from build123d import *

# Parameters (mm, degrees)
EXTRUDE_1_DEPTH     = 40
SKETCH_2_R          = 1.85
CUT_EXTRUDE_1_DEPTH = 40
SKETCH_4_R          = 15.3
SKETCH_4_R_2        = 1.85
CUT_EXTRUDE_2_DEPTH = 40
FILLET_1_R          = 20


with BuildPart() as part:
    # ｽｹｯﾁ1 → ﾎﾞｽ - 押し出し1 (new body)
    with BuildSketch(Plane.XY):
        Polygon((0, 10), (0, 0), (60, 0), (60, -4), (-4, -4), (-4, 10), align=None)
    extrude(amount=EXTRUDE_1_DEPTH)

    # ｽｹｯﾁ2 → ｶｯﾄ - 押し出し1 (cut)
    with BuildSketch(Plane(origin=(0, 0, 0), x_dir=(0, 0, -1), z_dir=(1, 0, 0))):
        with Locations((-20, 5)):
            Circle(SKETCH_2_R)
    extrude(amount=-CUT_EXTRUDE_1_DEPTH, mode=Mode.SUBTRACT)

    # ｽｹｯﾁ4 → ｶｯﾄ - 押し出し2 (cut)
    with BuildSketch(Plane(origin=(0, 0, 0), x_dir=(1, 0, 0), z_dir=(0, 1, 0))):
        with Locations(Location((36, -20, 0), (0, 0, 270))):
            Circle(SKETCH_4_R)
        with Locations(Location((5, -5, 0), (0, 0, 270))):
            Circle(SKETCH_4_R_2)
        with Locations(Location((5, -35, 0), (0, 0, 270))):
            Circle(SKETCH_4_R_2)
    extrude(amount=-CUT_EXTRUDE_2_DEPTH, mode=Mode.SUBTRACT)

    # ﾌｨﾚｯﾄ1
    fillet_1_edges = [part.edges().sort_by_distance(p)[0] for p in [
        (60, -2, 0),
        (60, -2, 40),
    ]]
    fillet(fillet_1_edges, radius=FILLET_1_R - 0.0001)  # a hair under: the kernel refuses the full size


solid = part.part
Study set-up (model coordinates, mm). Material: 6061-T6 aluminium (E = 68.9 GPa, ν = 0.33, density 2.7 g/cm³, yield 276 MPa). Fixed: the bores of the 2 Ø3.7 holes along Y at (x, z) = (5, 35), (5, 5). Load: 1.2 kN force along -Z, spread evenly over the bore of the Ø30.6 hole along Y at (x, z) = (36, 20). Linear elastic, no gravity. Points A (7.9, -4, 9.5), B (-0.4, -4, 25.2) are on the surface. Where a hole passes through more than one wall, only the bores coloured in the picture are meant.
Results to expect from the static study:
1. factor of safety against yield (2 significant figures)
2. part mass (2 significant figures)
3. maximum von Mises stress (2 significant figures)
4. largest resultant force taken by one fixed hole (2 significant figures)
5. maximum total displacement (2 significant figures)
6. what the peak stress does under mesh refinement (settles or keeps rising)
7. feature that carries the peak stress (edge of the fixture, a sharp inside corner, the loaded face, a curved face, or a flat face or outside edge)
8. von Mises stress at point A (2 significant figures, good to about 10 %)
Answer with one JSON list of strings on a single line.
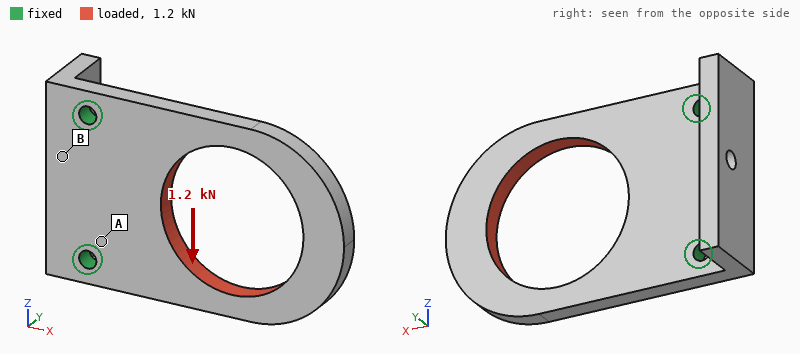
["2.5", "22 g", "110 MPa", "1.3 kN", "0.14 mm", "settles", "the loaded face", "21 MPa"]
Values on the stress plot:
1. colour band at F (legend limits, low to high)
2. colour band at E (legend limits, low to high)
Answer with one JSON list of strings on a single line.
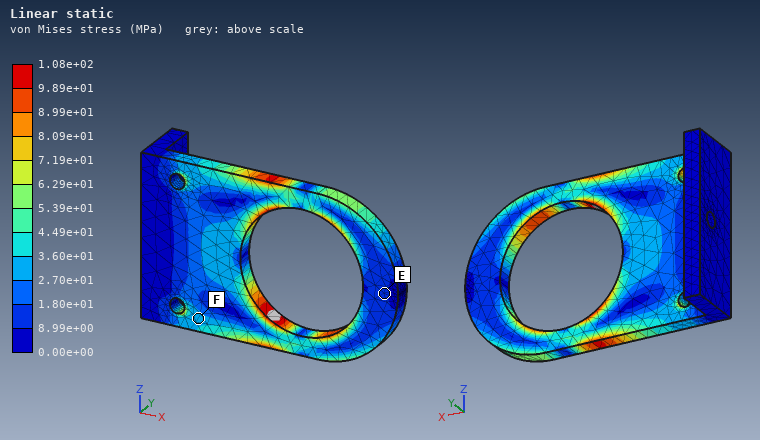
["2.70e+01 to 3.60e+01 MPa", "8.99e+00 to 1.80e+01 MPa"]
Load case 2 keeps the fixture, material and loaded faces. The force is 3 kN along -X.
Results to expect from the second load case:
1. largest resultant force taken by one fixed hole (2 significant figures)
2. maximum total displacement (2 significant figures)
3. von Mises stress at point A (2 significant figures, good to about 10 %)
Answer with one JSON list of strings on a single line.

["1.5 kN", "49 µm", "13 MPa"]
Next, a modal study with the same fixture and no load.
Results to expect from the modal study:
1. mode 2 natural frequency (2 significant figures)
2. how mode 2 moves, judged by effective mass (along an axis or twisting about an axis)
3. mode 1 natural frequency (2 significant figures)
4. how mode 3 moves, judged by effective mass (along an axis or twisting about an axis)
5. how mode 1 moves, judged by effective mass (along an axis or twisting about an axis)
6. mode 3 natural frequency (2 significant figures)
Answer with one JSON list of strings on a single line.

["3400 Hz", "twisting about X", "1200 Hz", "along Z", "along Y", "5300 Hz"]
